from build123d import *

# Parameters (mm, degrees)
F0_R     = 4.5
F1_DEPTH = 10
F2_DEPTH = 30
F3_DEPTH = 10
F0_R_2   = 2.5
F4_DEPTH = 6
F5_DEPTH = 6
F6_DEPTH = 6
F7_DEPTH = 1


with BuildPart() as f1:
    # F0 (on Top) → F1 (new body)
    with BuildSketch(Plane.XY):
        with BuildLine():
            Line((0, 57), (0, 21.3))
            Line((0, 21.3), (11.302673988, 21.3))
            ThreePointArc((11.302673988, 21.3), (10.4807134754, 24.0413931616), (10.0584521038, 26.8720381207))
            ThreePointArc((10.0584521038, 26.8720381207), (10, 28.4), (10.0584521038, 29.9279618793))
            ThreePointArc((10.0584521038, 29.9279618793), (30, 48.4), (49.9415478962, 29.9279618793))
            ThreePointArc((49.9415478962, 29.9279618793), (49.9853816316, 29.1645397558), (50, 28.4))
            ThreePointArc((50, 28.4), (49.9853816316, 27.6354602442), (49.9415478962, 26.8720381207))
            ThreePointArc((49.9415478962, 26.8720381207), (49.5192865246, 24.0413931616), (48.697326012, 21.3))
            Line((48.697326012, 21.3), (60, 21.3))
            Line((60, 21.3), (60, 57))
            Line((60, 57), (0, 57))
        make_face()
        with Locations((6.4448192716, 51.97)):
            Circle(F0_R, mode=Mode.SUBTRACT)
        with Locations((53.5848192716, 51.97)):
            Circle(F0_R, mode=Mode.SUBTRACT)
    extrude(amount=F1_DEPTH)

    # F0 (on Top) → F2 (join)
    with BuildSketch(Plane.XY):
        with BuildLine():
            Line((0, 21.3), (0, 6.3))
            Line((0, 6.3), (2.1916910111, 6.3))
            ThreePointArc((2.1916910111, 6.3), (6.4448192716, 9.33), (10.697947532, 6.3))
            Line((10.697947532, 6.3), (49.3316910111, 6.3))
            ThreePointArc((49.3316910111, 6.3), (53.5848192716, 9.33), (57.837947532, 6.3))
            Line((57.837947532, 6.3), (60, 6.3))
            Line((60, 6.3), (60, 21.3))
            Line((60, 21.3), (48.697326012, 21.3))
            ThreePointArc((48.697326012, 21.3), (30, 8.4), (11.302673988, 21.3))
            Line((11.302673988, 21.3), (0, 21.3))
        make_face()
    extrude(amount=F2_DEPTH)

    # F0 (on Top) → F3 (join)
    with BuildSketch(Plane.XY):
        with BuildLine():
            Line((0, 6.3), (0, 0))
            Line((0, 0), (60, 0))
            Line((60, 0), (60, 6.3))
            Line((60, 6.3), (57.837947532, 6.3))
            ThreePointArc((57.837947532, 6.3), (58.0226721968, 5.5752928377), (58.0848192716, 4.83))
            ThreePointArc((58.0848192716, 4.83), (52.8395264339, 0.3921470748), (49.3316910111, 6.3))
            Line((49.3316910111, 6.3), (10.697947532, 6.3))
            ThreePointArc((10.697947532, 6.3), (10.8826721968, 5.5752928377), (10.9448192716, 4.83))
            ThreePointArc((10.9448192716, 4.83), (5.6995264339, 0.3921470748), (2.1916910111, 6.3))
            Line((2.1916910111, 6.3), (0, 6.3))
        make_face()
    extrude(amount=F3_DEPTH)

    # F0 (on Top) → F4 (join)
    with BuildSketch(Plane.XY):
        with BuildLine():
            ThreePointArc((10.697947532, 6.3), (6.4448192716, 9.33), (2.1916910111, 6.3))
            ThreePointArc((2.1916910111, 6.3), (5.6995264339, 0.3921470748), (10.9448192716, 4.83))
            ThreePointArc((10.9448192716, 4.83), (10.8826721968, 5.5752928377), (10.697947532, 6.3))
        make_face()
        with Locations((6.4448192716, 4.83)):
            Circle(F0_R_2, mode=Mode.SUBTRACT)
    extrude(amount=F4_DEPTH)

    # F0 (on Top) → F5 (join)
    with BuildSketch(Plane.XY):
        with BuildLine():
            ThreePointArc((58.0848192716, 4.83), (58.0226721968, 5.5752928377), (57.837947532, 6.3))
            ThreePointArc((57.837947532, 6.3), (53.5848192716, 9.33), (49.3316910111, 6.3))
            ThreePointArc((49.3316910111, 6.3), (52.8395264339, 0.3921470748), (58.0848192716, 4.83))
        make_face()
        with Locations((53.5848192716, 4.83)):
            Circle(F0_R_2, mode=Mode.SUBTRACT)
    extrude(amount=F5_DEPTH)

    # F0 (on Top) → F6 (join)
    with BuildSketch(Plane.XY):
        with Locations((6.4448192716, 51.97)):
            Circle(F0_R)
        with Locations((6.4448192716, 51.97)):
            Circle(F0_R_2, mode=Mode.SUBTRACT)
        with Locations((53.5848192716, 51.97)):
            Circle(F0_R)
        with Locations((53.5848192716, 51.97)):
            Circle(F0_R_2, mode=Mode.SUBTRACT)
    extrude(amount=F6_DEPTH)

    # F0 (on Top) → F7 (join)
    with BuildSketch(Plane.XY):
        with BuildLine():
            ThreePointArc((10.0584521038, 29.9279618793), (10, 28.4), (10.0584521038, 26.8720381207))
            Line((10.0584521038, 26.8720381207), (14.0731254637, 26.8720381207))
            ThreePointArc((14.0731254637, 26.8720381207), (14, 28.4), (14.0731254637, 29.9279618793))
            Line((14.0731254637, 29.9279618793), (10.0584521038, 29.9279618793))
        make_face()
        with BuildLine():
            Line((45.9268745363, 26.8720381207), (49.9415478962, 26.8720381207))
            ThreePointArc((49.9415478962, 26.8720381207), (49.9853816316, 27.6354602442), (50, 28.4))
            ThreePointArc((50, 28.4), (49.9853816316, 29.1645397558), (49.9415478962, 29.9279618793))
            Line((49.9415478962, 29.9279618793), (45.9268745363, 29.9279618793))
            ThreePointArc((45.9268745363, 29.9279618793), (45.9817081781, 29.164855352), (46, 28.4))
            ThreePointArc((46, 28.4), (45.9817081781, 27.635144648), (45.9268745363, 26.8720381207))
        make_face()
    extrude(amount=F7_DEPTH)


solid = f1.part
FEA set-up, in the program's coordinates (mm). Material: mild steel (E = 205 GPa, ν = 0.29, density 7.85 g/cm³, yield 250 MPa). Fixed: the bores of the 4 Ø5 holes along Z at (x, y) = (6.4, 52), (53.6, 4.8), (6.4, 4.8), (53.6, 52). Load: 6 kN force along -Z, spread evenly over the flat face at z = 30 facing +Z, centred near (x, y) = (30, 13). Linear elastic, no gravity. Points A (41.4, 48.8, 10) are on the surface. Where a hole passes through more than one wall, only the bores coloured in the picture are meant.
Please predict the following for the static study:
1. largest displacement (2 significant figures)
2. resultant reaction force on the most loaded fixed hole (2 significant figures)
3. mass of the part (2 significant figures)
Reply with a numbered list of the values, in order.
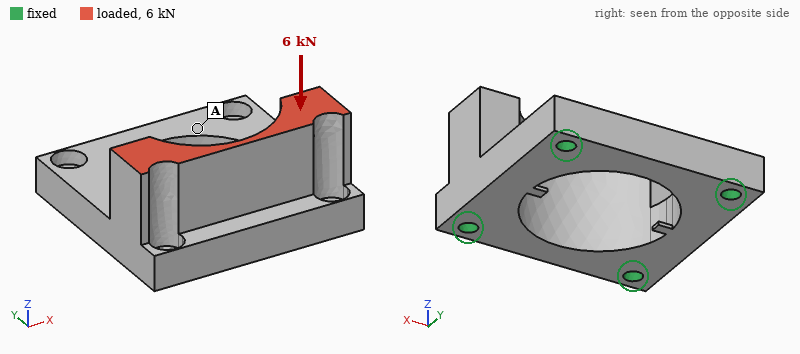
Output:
1. 9.7 µm
2. 2.7 kN
3. 240 g
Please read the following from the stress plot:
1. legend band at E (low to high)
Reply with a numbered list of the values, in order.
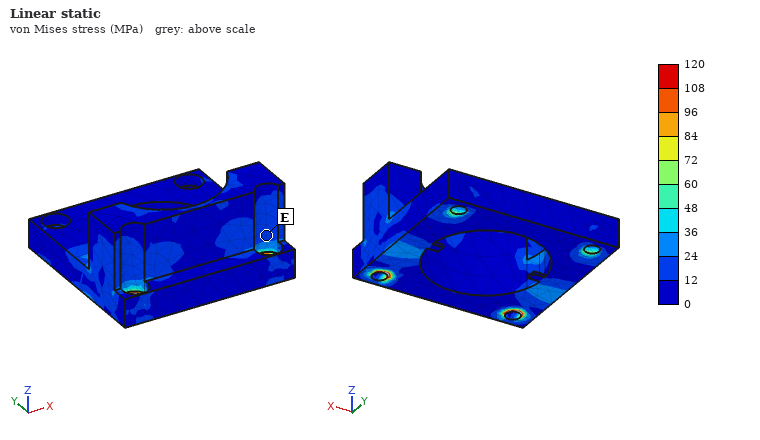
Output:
1. 12 to 24 MPa
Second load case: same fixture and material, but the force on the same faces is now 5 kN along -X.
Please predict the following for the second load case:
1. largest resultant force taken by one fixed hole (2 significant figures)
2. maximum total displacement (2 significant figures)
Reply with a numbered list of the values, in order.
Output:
1. 3.5 kN
2. 17 µm
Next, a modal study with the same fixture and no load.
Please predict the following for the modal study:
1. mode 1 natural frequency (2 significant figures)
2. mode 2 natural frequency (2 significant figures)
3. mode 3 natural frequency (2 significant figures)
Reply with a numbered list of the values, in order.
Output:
1. 8200 Hz
2. 9600 Hz
3. 12 kHz
